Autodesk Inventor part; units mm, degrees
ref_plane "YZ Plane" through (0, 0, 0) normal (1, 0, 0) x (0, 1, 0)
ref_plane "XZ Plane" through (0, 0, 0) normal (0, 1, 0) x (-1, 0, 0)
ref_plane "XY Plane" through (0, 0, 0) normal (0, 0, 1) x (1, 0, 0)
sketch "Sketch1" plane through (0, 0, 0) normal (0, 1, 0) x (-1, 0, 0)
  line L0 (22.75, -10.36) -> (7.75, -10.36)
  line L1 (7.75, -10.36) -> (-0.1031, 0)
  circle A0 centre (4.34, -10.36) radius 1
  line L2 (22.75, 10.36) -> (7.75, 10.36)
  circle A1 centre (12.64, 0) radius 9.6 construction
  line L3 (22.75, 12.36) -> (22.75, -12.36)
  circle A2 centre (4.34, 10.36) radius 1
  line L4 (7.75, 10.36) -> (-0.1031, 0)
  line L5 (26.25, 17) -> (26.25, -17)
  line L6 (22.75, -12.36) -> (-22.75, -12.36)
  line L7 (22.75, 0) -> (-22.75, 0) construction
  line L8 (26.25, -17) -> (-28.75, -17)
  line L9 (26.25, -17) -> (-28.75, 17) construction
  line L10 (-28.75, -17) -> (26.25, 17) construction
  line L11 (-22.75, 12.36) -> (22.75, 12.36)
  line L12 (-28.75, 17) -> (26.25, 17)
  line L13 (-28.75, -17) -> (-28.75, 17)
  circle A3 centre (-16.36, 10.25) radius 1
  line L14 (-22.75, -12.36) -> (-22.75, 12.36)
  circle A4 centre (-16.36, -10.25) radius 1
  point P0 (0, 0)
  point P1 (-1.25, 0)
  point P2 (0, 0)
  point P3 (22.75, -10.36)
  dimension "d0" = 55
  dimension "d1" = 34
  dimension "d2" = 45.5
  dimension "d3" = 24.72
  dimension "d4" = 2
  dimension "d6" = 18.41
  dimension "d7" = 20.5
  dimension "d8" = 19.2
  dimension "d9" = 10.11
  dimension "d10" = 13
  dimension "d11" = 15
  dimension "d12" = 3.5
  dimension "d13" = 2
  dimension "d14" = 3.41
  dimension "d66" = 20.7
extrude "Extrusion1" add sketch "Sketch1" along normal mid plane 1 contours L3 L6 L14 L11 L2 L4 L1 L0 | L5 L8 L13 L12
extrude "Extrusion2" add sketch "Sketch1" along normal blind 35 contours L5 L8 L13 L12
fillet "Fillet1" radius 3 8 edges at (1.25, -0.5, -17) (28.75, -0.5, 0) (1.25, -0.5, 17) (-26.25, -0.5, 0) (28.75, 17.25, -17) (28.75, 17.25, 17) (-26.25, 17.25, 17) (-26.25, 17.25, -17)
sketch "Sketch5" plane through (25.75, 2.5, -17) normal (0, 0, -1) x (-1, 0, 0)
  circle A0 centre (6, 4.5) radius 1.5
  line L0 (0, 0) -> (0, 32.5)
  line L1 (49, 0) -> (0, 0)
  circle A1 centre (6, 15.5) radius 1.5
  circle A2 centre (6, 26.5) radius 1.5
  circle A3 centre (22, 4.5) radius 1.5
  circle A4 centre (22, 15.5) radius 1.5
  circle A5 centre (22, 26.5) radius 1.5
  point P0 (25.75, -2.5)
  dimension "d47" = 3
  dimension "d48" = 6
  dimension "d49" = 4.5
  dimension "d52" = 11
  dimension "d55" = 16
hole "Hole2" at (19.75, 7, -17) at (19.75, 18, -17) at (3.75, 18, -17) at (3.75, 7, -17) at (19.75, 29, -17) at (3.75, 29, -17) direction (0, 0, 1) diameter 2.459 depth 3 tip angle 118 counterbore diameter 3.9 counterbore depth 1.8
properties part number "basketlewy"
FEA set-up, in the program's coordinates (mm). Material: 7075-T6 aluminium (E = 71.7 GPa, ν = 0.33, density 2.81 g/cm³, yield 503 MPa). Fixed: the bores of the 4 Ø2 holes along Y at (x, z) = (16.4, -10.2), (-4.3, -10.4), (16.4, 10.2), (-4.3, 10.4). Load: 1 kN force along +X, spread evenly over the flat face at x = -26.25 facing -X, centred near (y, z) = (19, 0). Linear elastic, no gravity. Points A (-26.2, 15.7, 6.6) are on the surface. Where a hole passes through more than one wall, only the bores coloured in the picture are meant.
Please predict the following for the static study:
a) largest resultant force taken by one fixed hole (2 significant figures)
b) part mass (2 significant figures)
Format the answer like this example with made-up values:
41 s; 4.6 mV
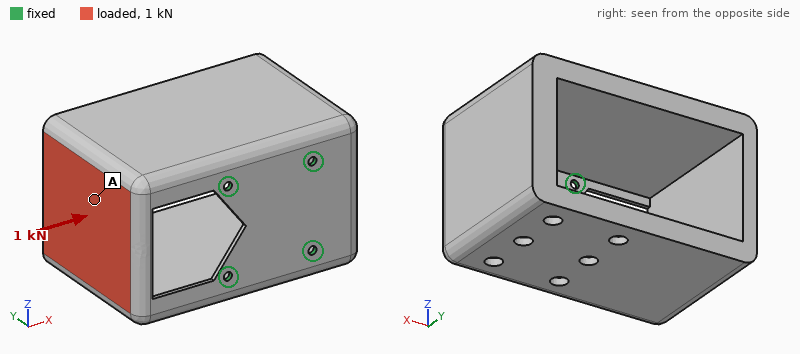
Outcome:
560 N; 74 g
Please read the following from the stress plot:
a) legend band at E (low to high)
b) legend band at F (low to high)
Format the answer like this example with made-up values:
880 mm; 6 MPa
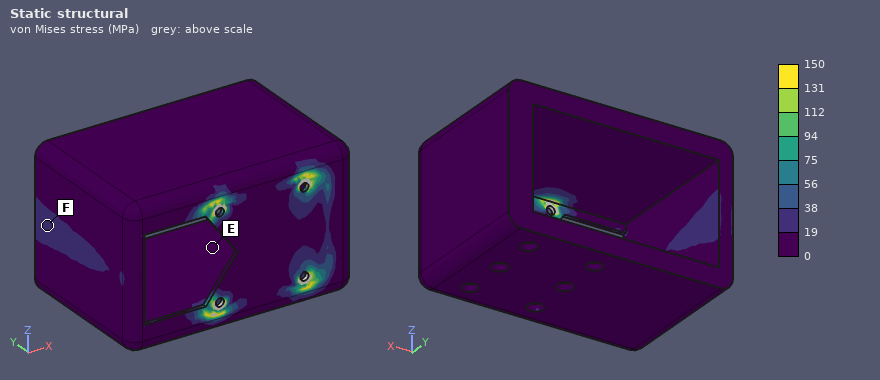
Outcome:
0 to 19 MPa; 19 to 38 MPa
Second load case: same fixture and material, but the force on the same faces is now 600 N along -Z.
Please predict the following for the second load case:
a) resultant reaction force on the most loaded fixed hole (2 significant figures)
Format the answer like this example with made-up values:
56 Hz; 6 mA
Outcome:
470 N
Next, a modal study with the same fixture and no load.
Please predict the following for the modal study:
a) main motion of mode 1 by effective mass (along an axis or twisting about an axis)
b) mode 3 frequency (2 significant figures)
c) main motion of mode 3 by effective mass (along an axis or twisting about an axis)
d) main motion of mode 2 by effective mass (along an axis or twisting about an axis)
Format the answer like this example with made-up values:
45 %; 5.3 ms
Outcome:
along Z; 4100 Hz; twisting about Y; along X
